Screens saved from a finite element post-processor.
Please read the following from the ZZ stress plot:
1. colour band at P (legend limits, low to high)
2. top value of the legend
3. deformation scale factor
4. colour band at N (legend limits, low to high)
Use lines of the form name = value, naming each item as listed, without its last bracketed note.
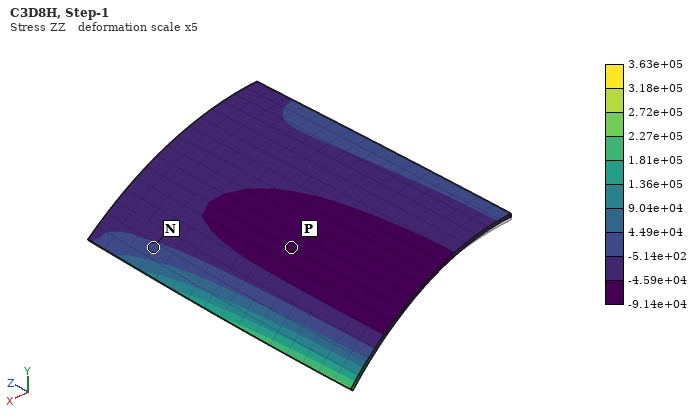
colour band at P = -9.14e+04 to -4.59e+04
top value of the legend = 3.63e+05
deformation scale factor = 5
colour band at N = -5.14e+02 to 4.49e+04
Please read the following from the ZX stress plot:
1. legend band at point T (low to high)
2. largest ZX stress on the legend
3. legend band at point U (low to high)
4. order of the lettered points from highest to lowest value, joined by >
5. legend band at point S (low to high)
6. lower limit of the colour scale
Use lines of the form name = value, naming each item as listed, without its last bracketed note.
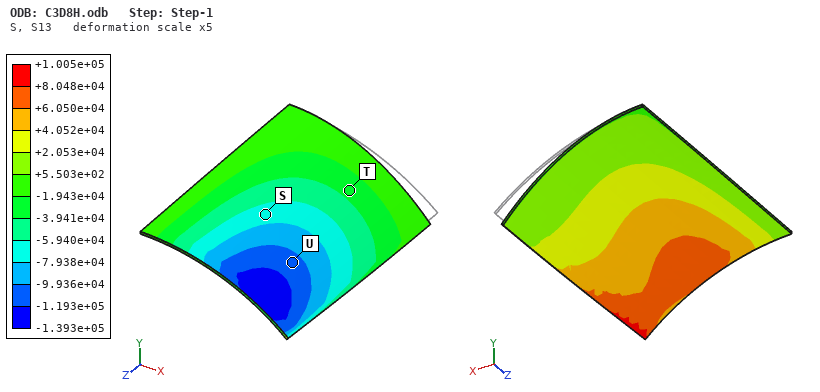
legend band at point T = -3.941e+04 to -1.943e+04
largest ZX stress on the legend = +1.005e+05
legend band at point U = -1.193e+05 to -9.936e+04
order of the lettered points from highest to lowest value, joined by > = T > S > U
legend band at point S = -7.938e+04 to -5.940e+04
lower limit of the colour scale = -1.393e+05
